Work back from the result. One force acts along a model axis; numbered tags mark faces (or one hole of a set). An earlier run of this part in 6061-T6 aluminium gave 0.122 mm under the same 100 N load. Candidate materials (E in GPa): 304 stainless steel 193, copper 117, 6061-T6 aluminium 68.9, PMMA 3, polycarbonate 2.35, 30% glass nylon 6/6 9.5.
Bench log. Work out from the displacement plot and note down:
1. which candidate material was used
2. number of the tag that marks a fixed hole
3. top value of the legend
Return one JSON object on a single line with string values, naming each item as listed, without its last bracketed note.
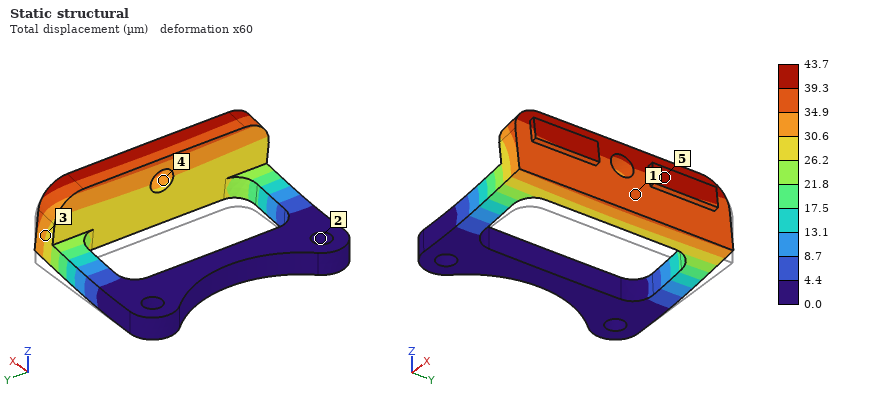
{"which candidate material was used": "304 stainless steel", "number of the tag that marks a fixed hole": "2", "top value of the legend": "43.7 µm"}
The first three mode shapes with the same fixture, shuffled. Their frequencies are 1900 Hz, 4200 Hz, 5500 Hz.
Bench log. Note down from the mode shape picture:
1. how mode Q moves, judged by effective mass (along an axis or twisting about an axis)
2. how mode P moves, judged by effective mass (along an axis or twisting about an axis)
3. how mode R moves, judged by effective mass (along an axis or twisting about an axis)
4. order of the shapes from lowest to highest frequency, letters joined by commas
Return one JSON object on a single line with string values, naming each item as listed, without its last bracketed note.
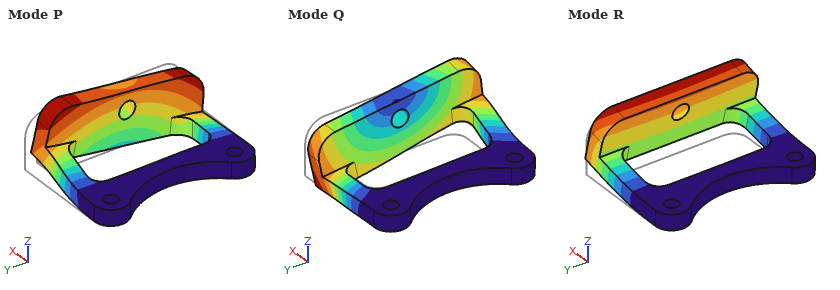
{"how mode Q moves, judged by effective mass": "along Y", "how mode P moves, judged by effective mass": "along Y", "how mode R moves, judged by effective mass": "along Z", "order of the shapes from lowest to highest frequency, letters joined by commas": "R, P, Q"}
